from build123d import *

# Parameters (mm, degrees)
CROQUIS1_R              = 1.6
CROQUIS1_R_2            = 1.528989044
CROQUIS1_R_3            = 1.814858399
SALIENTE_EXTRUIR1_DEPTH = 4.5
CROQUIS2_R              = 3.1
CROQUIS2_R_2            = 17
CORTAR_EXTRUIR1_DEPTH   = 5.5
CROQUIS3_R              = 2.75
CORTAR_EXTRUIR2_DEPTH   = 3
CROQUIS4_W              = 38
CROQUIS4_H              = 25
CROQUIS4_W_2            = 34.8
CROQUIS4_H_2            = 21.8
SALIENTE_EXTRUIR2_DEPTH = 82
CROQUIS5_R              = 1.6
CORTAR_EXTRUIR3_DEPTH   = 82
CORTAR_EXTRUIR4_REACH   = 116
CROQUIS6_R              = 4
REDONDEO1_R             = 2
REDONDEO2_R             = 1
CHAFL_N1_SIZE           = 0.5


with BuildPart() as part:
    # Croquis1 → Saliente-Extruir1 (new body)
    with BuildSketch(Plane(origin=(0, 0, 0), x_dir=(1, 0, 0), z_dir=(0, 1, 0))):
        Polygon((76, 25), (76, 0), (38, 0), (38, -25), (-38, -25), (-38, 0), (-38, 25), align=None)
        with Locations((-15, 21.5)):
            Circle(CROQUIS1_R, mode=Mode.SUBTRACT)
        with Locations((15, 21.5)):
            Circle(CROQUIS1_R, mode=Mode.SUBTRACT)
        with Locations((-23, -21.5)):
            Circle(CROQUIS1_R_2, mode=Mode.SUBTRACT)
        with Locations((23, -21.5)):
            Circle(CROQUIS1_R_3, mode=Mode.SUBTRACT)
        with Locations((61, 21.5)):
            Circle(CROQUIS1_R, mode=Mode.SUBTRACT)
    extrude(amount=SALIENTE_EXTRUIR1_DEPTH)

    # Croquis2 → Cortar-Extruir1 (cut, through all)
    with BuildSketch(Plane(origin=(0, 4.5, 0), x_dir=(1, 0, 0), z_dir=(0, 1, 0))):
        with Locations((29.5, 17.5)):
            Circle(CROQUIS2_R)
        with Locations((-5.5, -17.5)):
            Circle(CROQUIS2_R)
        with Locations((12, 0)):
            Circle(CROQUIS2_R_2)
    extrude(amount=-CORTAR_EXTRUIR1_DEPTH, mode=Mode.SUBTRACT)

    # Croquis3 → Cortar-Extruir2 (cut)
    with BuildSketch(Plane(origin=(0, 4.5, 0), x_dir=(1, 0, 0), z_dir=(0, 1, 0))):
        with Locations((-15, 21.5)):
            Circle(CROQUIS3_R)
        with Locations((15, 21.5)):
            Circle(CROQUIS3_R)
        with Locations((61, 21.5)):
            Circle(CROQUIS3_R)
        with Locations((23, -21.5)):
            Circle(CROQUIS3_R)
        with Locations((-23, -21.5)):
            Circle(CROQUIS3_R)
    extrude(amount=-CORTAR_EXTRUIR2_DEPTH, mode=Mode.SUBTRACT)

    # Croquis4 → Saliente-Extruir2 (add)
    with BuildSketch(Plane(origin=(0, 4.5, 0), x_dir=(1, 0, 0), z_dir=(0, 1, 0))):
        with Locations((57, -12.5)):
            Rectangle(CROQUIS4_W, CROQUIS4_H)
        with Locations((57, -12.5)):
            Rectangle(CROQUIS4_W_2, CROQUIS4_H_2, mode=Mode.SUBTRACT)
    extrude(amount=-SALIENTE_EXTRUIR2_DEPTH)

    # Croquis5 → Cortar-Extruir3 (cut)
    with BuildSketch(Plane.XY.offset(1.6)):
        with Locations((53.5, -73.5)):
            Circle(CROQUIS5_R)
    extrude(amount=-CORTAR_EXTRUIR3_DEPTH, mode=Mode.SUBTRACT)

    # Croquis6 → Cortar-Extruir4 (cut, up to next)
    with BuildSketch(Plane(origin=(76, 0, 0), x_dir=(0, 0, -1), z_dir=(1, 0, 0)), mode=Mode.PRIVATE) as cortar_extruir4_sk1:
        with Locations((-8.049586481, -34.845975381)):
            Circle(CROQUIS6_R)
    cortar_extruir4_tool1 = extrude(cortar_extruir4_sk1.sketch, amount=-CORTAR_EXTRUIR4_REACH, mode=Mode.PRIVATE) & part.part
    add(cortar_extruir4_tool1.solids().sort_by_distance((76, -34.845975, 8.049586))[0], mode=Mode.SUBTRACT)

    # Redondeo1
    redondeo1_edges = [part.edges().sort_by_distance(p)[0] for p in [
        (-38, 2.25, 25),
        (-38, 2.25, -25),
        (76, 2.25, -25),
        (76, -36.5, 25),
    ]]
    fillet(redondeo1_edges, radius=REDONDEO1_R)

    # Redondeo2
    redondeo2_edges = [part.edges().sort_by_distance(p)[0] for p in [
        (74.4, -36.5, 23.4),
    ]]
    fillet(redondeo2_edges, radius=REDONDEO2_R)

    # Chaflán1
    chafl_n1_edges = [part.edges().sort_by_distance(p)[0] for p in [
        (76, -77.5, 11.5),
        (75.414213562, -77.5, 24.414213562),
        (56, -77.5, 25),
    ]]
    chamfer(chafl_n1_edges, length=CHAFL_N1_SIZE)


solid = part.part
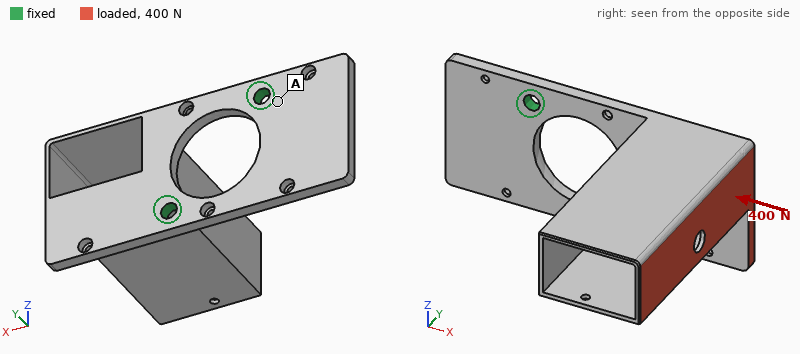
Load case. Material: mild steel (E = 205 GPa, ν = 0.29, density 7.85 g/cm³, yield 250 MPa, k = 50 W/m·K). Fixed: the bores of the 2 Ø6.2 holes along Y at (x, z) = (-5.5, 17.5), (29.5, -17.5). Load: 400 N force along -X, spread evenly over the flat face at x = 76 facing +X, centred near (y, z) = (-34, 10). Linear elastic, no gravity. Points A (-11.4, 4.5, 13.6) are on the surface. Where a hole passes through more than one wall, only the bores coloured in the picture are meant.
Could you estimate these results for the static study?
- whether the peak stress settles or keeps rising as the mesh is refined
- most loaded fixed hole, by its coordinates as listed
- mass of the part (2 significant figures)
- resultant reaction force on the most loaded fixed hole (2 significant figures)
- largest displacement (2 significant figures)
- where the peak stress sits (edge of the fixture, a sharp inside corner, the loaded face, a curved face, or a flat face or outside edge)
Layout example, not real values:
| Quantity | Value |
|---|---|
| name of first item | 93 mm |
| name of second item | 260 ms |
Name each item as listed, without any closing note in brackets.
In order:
| Quantity | Value |
|---|---|
| whether the peak stress settles or keeps rising as the mesh is refined | keeps rising |
| most loaded fixed hole, by its coordinates as listed | (-5.5, 17.5) |
| mass of the part | 250 g |
| resultant reaction force on the most loaded fixed hole | 280 N |
| largest displacement | 0.53 mm |
| where the peak stress sits | edge of the fixture |
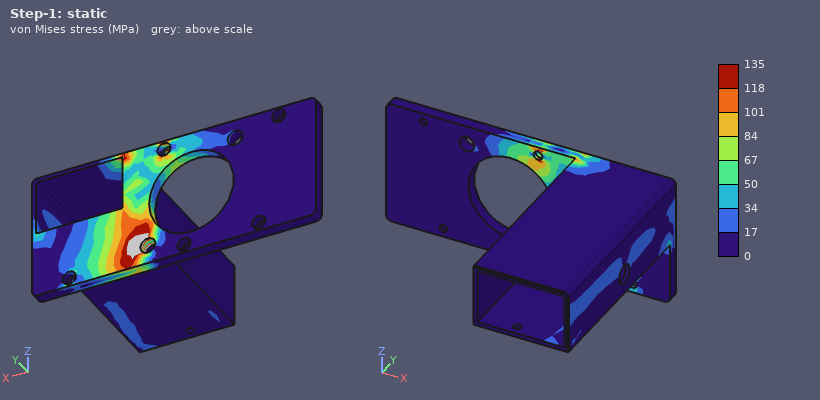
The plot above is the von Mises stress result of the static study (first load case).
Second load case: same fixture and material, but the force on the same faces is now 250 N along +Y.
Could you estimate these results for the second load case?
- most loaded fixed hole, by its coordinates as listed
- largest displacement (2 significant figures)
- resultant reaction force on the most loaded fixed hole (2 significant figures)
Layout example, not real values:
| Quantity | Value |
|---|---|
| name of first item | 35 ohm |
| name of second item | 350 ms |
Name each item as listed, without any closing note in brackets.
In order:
| Quantity | Value |
|---|---|
| most loaded fixed hole, by its coordinates as listed | (29.5, -17.5) |
| largest displacement | 0.46 mm |
| resultant reaction force on the most loaded fixed hole | 260 N |
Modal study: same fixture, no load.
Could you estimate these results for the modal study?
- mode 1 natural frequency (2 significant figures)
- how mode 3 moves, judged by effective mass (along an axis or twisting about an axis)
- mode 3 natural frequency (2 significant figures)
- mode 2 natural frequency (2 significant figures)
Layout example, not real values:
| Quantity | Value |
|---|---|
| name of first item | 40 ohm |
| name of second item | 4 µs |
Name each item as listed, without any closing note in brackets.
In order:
| Quantity | Value |
|---|---|
| mode 1 natural frequency | 380 Hz |
| how mode 3 moves, judged by effective mass | along Y |
| mode 3 natural frequency | 1700 Hz |
| mode 2 natural frequency | 600 Hz |
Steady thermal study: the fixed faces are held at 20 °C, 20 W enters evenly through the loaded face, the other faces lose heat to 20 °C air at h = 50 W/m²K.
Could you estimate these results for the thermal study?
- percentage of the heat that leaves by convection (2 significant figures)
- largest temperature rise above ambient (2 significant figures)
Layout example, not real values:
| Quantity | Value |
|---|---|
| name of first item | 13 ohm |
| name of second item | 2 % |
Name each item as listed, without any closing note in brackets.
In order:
| Quantity | Value |
|---|---|
| percentage of the heat that leaves by convection | 89 % |
| largest temperature rise above ambient | 40 K |
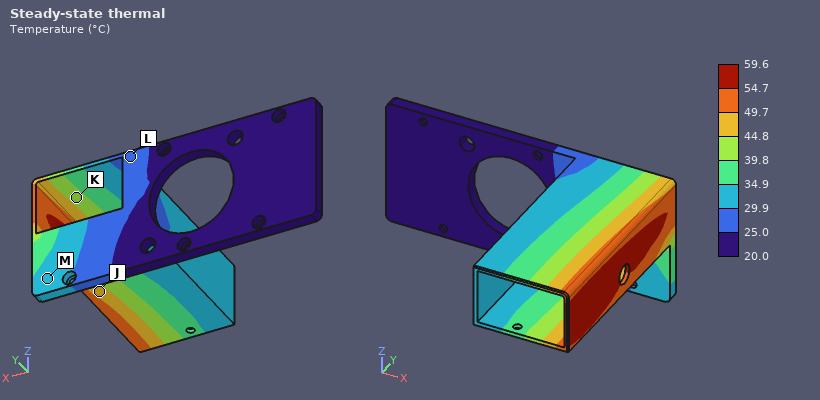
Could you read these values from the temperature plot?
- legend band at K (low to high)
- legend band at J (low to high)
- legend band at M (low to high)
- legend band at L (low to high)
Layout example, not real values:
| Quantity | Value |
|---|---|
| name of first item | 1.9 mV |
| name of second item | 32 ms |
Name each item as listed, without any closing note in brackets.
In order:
| Quantity | Value |
|---|---|
| legend band at K | 39.8 to 44.8 °C |
| legend band at J | 44.8 to 49.7 °C |
| legend band at M | 29.9 to 34.9 °C |
| legend band at L | 25.0 to 29.9 °C |
